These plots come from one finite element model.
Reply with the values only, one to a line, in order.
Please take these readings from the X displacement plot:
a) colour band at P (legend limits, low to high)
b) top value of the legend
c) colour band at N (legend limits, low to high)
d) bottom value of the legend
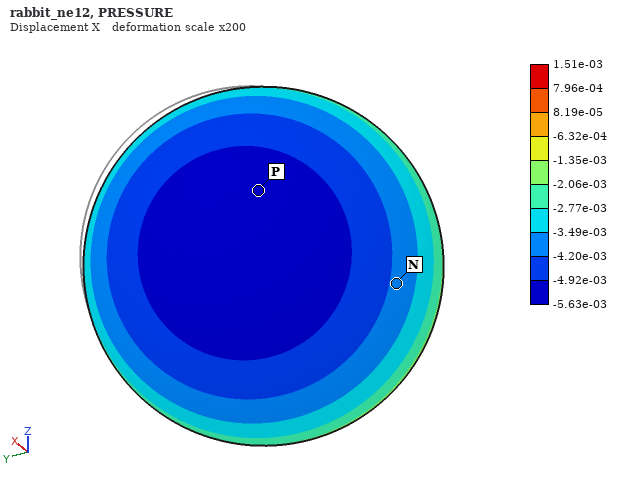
-5.63e-03 to -4.92e-03
1.51e-03
-4.20e-03 to -3.49e-03
-5.63e-03
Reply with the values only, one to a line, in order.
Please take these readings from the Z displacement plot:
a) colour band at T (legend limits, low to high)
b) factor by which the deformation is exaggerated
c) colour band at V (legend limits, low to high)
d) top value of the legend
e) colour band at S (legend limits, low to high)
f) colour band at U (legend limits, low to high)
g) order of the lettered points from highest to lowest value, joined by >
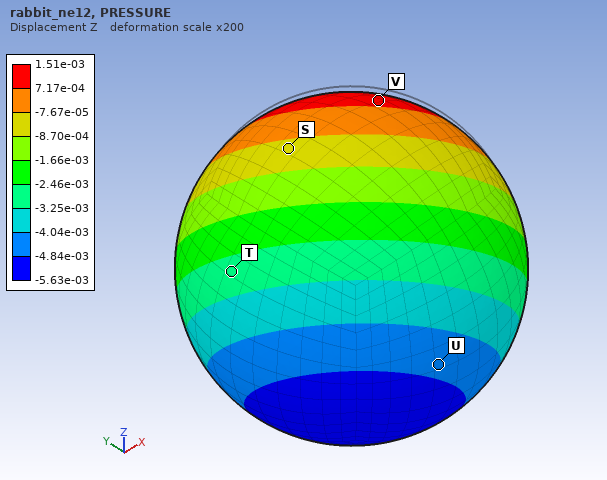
-3.25e-03 to -2.46e-03
200
7.17e-04 to 1.51e-03
1.51e-03
-8.70e-04 to -7.67e-05
-4.84e-03 to -4.04e-03
V > S > T > U
